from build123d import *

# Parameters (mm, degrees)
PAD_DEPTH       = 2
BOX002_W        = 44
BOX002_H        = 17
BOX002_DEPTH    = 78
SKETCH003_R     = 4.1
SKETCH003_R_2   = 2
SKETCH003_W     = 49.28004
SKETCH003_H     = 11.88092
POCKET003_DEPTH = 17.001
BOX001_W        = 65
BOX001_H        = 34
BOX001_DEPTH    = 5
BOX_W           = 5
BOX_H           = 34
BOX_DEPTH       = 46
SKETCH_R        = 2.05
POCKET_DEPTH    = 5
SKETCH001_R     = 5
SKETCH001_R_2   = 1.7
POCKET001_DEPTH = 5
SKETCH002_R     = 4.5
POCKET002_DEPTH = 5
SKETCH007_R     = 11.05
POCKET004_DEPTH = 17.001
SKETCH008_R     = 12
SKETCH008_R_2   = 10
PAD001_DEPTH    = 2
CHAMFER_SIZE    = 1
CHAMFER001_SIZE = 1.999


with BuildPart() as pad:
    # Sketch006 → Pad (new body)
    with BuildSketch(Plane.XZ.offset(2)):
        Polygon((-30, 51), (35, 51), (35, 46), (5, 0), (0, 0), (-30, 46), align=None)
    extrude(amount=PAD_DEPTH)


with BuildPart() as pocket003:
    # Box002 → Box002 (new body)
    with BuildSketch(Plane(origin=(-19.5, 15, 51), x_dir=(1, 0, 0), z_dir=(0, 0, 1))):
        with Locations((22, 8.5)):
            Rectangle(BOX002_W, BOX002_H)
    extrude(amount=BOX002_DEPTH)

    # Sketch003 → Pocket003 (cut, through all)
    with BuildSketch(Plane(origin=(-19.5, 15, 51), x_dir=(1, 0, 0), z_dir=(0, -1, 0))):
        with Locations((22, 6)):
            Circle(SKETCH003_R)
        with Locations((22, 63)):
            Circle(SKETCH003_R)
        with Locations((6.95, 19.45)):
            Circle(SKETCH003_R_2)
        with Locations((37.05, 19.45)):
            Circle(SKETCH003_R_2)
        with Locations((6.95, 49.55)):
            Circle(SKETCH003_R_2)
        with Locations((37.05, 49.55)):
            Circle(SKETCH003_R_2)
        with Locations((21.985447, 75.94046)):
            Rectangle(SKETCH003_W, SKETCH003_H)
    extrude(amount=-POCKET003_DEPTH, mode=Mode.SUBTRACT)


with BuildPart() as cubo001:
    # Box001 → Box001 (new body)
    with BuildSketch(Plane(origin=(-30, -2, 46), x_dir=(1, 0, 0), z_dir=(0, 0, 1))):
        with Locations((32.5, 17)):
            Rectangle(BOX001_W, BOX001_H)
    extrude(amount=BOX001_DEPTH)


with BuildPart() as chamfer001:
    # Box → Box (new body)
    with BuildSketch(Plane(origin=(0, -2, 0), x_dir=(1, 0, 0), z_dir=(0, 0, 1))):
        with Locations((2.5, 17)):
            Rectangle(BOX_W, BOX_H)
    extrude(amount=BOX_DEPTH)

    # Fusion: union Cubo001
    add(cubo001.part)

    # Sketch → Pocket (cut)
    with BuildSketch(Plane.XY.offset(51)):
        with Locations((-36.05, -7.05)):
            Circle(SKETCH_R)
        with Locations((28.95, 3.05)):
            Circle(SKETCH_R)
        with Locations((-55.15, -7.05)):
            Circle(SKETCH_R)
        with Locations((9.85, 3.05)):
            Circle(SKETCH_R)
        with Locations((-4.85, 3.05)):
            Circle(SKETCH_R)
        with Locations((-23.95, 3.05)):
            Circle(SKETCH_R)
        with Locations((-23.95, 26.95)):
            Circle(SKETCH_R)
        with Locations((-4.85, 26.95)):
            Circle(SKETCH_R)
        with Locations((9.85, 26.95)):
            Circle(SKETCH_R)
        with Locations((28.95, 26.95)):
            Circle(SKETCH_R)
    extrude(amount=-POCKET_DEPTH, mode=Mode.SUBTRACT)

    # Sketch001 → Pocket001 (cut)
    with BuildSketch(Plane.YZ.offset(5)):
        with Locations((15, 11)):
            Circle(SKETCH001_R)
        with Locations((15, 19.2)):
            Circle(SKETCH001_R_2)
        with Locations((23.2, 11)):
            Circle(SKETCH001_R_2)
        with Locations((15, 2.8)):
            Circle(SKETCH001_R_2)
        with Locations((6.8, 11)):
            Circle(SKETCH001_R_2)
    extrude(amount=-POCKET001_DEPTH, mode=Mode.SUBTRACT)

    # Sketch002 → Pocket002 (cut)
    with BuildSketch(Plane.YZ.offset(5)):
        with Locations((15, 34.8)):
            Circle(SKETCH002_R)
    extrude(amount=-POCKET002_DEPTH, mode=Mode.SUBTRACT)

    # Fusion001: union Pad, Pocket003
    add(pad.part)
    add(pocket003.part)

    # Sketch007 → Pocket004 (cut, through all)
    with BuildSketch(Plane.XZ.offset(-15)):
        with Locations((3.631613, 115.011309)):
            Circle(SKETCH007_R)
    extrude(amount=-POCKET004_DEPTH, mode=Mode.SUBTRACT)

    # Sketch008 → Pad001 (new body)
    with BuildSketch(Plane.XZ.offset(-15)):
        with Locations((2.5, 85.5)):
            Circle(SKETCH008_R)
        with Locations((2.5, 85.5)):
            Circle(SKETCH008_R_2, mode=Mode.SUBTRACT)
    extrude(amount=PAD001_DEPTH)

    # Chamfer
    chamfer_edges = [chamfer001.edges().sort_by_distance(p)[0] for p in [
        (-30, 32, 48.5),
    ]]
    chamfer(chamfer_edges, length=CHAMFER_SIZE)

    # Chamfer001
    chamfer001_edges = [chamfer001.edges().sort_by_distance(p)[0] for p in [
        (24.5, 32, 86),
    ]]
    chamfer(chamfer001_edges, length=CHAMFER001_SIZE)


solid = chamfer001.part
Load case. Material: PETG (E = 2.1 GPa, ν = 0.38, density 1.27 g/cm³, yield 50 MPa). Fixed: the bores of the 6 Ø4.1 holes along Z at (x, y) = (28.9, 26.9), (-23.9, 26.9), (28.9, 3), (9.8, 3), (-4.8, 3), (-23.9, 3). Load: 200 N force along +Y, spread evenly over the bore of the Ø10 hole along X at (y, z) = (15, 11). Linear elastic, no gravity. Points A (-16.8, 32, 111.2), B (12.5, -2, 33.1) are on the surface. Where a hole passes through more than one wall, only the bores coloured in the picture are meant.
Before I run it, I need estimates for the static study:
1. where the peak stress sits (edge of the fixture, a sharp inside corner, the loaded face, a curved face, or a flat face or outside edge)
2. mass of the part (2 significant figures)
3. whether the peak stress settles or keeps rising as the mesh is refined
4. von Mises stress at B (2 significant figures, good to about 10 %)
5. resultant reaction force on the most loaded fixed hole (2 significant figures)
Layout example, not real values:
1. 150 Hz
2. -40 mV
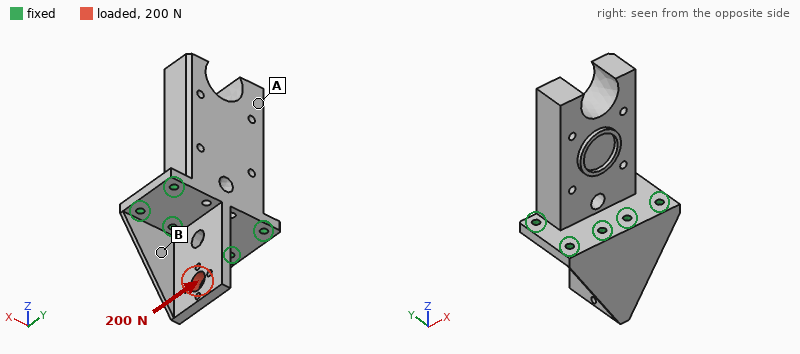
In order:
1. edge of the fixture
2. 85 g
3. keeps rising
4. 1.9 MPa
5. 140 N
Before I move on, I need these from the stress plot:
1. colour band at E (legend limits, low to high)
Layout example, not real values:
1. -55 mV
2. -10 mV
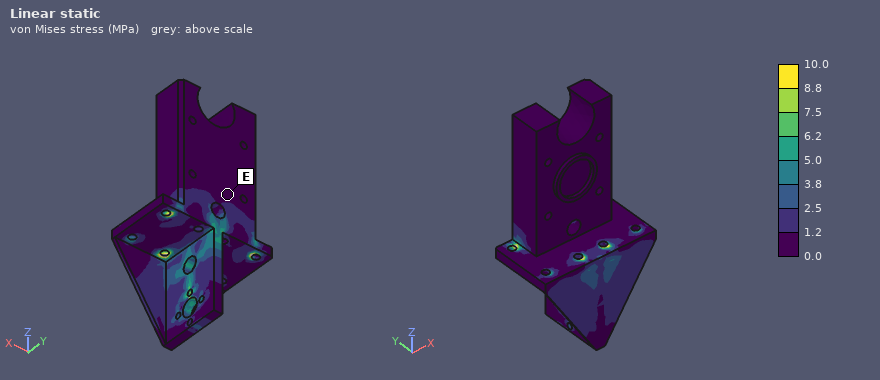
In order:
1. 0.0 to 1.2 MPa
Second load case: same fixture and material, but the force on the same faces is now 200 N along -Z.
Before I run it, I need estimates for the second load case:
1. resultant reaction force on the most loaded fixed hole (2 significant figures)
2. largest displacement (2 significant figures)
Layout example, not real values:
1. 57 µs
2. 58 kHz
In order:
1. 52 N
2. 70 µm
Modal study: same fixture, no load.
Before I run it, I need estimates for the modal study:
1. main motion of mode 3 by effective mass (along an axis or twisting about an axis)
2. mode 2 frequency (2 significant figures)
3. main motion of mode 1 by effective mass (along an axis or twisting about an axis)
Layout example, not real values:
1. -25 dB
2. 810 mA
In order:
1. along X
2. 790 Hz
3. along Y
